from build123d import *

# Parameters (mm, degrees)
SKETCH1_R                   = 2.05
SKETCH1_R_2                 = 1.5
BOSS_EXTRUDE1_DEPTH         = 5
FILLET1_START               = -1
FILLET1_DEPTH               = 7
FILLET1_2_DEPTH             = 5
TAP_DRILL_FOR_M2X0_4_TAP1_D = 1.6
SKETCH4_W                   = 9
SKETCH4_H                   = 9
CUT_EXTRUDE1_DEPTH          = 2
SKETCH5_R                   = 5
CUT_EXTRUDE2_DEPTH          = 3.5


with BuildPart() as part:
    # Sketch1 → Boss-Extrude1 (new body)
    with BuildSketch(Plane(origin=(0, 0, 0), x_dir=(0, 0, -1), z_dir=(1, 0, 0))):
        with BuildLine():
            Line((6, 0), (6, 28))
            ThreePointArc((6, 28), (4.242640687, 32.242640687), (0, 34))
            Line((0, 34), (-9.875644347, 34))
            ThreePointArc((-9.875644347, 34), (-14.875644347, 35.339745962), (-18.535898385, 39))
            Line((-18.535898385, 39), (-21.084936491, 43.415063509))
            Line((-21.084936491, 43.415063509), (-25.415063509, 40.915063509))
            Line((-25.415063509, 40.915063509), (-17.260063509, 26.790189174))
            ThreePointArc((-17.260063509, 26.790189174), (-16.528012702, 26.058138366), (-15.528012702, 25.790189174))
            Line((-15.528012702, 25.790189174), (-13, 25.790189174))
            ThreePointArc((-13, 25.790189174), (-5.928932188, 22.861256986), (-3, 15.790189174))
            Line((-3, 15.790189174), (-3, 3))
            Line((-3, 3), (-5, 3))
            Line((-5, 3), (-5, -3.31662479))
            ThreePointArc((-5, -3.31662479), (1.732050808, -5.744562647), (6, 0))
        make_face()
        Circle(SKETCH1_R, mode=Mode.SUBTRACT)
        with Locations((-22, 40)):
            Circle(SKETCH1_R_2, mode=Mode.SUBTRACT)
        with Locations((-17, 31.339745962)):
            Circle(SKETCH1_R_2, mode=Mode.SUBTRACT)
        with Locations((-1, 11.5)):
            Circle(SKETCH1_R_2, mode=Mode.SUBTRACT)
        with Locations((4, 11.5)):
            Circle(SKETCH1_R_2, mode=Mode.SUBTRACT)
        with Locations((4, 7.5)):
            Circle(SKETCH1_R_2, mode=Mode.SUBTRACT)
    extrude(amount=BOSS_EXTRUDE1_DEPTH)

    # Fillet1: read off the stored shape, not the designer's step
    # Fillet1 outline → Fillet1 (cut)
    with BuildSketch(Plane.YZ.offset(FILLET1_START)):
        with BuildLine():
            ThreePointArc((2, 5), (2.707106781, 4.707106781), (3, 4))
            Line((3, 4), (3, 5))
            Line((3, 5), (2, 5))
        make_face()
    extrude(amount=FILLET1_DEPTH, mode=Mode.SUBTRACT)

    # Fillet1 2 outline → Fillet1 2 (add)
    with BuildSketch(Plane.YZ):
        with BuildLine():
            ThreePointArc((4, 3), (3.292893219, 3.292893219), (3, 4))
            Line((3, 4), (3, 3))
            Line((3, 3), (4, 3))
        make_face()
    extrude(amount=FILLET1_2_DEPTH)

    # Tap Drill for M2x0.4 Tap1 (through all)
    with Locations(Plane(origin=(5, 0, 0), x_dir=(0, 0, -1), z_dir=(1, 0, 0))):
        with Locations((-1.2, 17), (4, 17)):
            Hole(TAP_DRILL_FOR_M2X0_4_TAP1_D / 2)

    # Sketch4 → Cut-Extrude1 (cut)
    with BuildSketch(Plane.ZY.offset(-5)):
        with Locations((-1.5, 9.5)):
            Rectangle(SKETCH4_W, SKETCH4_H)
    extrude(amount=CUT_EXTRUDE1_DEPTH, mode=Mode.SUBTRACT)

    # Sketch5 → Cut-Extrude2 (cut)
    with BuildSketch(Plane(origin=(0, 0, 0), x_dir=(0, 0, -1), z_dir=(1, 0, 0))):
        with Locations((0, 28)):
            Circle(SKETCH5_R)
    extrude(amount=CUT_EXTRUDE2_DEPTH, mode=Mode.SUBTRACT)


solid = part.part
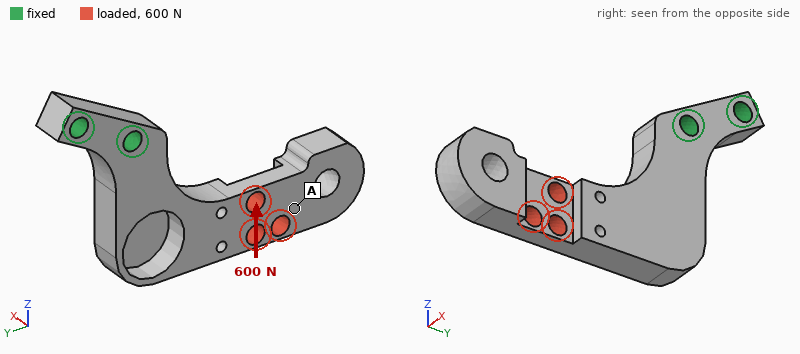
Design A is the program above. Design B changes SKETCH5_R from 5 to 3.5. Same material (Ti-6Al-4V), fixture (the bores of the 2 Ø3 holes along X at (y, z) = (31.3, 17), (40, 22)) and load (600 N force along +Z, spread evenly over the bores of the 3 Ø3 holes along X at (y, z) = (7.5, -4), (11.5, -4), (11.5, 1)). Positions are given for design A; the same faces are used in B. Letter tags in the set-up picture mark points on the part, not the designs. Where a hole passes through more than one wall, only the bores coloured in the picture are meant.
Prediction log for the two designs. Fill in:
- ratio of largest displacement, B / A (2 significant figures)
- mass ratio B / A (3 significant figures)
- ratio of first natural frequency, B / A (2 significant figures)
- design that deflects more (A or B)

0.88
1.06
1.1
A
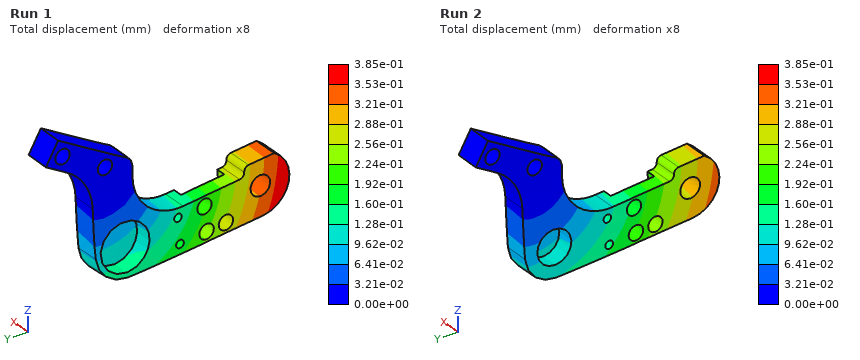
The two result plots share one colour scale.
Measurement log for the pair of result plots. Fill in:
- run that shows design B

Run 2
